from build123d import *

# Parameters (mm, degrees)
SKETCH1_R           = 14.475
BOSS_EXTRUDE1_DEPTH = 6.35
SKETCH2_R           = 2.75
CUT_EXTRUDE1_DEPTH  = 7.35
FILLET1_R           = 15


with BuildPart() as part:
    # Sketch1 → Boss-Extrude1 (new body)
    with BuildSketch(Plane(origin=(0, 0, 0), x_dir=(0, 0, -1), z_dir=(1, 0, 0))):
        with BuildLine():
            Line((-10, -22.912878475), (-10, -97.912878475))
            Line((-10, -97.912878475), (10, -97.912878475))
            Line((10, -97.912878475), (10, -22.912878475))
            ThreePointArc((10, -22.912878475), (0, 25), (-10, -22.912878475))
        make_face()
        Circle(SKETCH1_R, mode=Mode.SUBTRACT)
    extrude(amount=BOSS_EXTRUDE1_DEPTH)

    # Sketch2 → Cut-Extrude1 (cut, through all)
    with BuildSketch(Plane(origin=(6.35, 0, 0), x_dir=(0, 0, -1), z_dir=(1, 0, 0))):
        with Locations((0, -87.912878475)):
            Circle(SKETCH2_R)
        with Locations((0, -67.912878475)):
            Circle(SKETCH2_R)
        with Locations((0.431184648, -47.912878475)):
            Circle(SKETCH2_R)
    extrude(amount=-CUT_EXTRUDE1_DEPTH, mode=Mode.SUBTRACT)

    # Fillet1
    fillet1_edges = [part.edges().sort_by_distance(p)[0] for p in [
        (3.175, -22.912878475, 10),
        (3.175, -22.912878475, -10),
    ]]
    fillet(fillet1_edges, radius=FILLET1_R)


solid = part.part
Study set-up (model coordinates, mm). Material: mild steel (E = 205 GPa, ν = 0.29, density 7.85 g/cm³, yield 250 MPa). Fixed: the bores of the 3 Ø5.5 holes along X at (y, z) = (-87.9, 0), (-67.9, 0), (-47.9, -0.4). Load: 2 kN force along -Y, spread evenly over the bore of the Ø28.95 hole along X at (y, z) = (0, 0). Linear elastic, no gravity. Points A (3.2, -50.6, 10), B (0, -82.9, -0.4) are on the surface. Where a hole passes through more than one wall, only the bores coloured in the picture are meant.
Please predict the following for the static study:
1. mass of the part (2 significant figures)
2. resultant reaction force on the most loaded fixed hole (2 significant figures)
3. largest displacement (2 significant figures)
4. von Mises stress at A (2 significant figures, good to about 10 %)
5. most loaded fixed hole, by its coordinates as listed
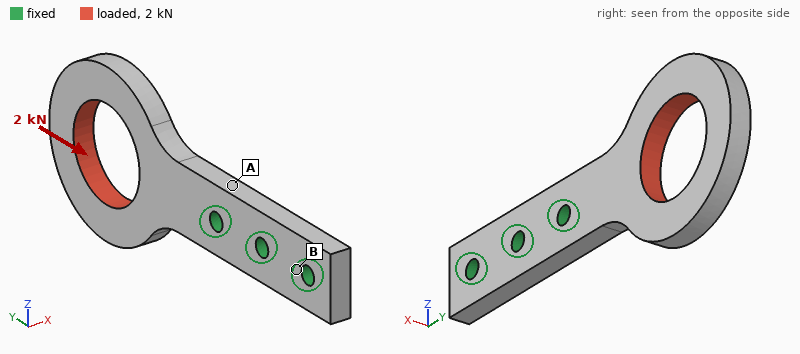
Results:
140 g
1.7 kN
9.4 µm
9.0 MPa
(-47.9, -0.4)
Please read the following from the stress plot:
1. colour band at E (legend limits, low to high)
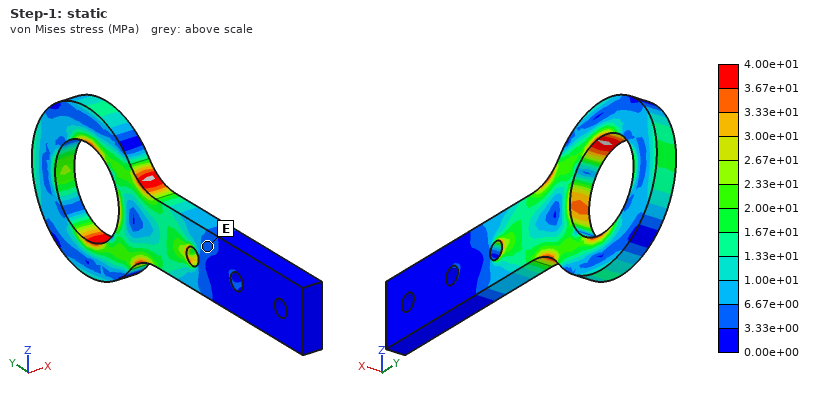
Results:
3.33e+00 to 6.67e+00 MPa
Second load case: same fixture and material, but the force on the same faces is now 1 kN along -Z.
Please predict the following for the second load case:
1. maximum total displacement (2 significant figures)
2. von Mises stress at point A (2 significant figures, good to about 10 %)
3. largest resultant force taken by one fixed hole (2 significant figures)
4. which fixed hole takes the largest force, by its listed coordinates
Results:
0.12 mm
75 MPa
2.3 kN
(-47.9, -0.4)
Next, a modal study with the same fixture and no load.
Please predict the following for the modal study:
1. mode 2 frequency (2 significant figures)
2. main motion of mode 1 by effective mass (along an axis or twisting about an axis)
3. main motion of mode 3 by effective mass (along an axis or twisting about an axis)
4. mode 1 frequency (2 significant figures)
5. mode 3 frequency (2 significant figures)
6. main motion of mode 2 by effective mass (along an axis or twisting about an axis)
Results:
2100 Hz
along X
twisting about Y
870 Hz
2300 Hz
along Z
